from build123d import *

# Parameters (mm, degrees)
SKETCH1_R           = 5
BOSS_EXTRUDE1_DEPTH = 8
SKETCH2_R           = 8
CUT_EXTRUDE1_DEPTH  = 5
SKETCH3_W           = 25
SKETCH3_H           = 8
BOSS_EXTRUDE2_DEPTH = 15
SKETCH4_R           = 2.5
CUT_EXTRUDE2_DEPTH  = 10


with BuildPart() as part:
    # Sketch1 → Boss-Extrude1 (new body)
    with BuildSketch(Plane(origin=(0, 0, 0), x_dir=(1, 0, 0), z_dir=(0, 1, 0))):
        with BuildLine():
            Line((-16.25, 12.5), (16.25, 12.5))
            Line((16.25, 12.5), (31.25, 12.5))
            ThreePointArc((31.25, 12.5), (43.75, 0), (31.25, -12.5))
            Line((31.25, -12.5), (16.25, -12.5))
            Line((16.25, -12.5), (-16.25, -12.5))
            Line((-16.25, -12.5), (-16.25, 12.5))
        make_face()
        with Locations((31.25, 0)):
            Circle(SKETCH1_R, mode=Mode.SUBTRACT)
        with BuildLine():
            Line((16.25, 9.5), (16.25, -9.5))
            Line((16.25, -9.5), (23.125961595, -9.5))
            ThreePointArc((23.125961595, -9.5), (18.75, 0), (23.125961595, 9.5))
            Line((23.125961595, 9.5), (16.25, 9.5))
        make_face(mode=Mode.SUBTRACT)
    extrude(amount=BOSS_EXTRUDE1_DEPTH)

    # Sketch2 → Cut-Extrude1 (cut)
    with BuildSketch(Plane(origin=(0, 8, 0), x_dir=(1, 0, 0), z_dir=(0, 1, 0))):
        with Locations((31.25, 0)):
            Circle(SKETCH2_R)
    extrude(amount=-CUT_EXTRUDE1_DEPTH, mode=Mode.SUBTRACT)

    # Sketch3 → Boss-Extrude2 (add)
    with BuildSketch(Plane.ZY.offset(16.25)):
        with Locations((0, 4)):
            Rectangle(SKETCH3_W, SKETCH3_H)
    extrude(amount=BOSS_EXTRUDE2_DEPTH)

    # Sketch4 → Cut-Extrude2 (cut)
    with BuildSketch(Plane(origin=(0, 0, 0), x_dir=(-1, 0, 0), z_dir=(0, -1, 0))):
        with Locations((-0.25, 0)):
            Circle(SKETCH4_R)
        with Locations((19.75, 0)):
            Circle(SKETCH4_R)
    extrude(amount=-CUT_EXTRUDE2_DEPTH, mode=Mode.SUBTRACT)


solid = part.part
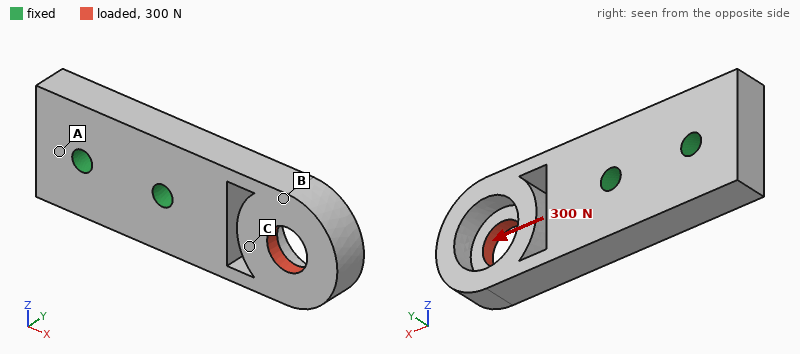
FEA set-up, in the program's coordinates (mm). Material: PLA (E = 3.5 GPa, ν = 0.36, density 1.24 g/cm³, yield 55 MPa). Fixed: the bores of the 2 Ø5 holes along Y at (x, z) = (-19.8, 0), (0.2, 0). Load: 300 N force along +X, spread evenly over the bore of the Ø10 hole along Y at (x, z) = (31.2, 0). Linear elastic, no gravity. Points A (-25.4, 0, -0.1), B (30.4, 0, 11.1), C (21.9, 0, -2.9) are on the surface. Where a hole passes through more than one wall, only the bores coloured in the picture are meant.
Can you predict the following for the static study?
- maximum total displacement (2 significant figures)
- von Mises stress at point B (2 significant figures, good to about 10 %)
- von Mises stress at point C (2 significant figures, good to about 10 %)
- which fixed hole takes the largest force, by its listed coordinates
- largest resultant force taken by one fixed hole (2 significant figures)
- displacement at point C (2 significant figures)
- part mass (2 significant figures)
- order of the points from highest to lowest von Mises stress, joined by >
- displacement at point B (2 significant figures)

0.42 mm
5.9 MPa
3.7 MPa
(0.2, 0)
230 N
0.13 mm
15 g
B > C > A
0.21 mm
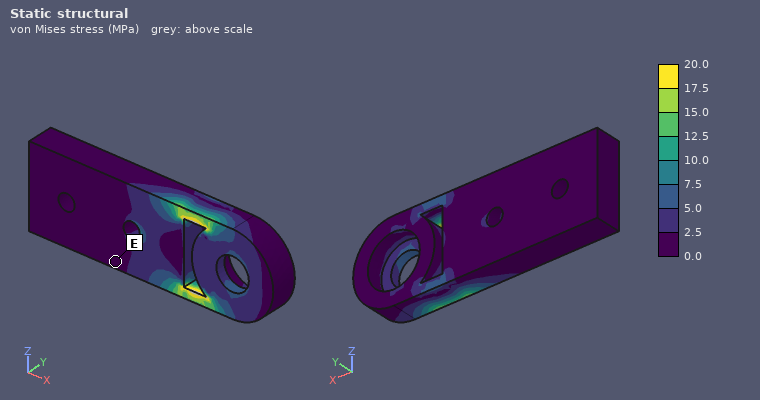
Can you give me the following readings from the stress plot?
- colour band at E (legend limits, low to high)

0.0 to 2.5 MPa
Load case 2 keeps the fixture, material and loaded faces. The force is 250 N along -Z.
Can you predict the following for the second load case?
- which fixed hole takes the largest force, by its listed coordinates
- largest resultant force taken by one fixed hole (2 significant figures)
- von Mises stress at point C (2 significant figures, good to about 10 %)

(0.2, 0)
510 N
3.9 MPa
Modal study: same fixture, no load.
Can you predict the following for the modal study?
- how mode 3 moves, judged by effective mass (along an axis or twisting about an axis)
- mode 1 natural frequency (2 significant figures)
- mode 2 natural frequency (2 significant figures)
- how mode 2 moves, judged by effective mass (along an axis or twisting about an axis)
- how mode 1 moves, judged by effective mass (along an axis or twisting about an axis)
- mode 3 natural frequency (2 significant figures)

twisting about X
1100 Hz
2000 Hz
along Z
along Y
3000 Hz
